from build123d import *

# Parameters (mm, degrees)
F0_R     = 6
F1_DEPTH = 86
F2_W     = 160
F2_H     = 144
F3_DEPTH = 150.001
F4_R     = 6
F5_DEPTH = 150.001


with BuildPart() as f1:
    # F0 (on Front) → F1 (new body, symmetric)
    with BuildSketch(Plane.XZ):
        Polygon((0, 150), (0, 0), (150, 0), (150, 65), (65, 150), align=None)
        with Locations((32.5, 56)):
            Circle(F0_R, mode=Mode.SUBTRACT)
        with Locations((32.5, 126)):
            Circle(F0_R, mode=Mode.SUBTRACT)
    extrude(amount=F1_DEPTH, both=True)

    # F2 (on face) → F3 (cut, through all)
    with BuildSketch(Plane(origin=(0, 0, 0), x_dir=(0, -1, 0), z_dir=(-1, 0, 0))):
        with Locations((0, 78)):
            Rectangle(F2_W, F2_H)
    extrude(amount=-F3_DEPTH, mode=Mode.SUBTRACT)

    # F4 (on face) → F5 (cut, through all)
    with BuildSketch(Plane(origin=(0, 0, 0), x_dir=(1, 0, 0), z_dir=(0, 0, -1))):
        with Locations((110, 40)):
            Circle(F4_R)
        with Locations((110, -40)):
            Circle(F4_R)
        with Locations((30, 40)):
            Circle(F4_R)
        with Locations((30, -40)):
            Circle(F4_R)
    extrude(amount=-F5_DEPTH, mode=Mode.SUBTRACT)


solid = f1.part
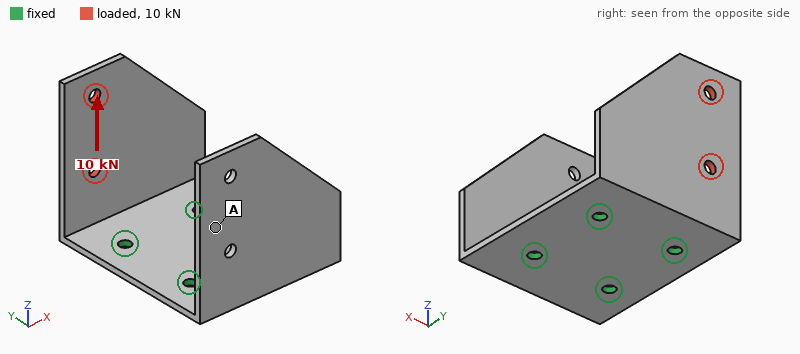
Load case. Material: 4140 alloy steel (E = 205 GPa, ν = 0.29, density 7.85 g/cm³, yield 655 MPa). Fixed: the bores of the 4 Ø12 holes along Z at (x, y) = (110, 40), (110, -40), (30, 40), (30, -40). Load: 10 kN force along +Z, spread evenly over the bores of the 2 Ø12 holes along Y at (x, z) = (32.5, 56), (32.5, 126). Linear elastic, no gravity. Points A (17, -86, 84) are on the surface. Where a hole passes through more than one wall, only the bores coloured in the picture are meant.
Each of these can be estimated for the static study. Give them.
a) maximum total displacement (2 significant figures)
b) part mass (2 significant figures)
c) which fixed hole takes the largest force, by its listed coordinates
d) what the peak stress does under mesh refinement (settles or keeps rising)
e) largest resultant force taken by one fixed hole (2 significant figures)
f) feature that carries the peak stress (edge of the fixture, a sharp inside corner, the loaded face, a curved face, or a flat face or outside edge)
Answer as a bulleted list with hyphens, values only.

- 2.9 mm
- 2.9 kg
- (30, 40)
- keeps rising
- 9.6 kN
- edge of the fixture
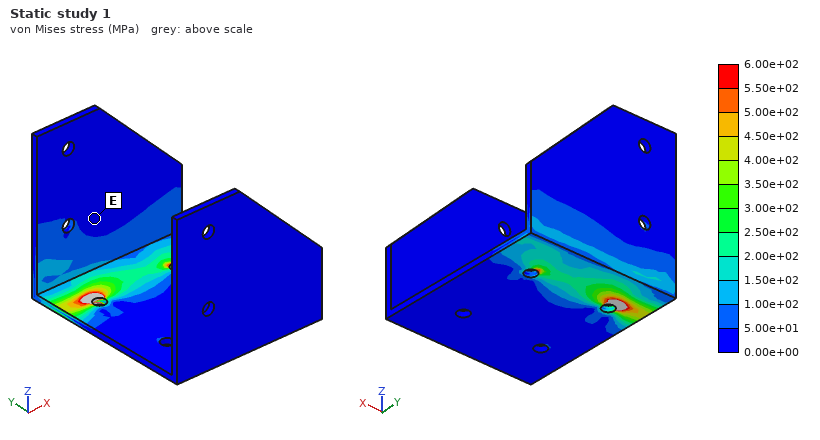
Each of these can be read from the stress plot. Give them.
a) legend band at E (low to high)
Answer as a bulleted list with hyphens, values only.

- 0.00e+00 to 5.00e+01 MPa
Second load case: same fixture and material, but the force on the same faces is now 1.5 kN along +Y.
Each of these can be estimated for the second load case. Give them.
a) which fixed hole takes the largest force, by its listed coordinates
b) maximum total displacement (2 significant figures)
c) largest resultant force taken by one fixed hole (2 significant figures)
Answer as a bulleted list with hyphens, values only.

- (30, 40)
- 3.1 mm
- 1.1 kN
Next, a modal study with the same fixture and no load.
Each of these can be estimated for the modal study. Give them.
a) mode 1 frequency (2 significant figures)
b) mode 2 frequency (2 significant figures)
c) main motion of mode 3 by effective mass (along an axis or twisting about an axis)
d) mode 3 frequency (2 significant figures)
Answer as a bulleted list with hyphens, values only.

- 200 Hz
- 200 Hz
- along X
- 520 Hz
